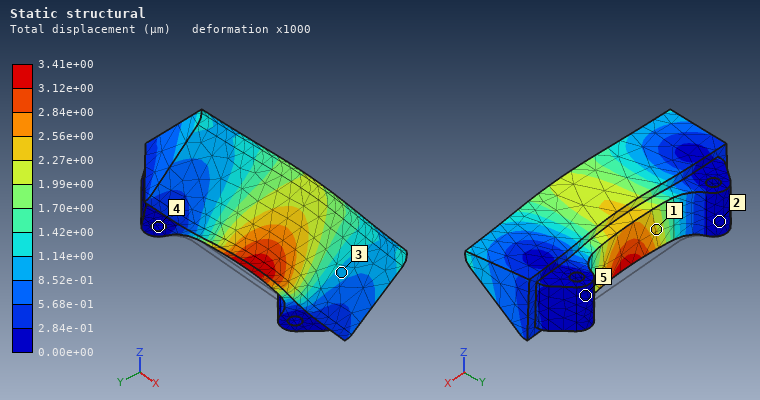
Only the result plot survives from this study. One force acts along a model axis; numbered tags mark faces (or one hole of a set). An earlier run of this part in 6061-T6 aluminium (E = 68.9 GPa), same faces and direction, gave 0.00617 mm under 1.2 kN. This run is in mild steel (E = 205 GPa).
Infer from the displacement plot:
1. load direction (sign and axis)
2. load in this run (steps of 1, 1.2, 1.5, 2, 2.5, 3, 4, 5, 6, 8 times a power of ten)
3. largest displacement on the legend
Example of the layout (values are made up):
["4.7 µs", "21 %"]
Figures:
["-Y", "2 kN", "3.41e+00 µm"]
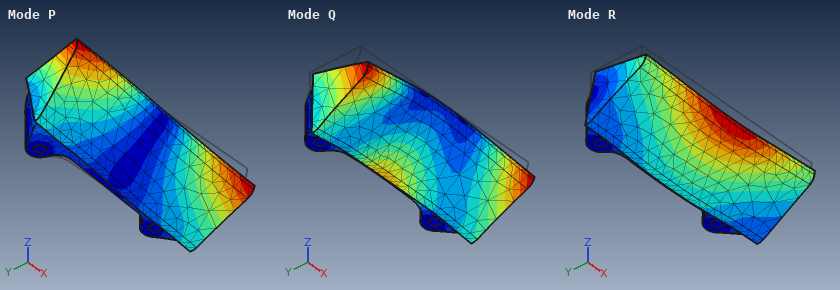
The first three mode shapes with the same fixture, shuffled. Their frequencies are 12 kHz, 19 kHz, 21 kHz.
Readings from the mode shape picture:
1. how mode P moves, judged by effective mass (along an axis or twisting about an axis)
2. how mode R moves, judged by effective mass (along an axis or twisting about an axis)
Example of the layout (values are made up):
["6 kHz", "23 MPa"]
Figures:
["twisting about Y", "along Z"]
